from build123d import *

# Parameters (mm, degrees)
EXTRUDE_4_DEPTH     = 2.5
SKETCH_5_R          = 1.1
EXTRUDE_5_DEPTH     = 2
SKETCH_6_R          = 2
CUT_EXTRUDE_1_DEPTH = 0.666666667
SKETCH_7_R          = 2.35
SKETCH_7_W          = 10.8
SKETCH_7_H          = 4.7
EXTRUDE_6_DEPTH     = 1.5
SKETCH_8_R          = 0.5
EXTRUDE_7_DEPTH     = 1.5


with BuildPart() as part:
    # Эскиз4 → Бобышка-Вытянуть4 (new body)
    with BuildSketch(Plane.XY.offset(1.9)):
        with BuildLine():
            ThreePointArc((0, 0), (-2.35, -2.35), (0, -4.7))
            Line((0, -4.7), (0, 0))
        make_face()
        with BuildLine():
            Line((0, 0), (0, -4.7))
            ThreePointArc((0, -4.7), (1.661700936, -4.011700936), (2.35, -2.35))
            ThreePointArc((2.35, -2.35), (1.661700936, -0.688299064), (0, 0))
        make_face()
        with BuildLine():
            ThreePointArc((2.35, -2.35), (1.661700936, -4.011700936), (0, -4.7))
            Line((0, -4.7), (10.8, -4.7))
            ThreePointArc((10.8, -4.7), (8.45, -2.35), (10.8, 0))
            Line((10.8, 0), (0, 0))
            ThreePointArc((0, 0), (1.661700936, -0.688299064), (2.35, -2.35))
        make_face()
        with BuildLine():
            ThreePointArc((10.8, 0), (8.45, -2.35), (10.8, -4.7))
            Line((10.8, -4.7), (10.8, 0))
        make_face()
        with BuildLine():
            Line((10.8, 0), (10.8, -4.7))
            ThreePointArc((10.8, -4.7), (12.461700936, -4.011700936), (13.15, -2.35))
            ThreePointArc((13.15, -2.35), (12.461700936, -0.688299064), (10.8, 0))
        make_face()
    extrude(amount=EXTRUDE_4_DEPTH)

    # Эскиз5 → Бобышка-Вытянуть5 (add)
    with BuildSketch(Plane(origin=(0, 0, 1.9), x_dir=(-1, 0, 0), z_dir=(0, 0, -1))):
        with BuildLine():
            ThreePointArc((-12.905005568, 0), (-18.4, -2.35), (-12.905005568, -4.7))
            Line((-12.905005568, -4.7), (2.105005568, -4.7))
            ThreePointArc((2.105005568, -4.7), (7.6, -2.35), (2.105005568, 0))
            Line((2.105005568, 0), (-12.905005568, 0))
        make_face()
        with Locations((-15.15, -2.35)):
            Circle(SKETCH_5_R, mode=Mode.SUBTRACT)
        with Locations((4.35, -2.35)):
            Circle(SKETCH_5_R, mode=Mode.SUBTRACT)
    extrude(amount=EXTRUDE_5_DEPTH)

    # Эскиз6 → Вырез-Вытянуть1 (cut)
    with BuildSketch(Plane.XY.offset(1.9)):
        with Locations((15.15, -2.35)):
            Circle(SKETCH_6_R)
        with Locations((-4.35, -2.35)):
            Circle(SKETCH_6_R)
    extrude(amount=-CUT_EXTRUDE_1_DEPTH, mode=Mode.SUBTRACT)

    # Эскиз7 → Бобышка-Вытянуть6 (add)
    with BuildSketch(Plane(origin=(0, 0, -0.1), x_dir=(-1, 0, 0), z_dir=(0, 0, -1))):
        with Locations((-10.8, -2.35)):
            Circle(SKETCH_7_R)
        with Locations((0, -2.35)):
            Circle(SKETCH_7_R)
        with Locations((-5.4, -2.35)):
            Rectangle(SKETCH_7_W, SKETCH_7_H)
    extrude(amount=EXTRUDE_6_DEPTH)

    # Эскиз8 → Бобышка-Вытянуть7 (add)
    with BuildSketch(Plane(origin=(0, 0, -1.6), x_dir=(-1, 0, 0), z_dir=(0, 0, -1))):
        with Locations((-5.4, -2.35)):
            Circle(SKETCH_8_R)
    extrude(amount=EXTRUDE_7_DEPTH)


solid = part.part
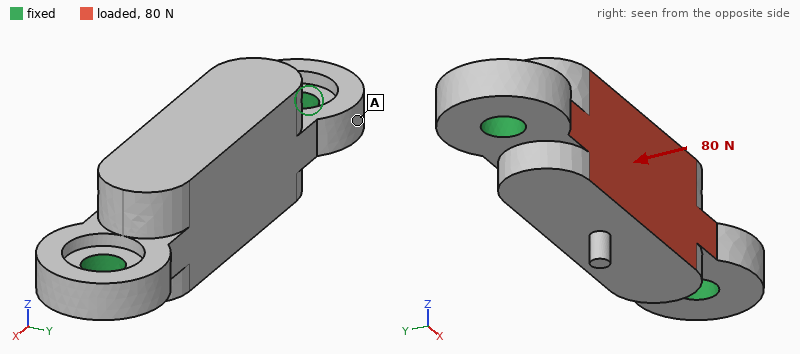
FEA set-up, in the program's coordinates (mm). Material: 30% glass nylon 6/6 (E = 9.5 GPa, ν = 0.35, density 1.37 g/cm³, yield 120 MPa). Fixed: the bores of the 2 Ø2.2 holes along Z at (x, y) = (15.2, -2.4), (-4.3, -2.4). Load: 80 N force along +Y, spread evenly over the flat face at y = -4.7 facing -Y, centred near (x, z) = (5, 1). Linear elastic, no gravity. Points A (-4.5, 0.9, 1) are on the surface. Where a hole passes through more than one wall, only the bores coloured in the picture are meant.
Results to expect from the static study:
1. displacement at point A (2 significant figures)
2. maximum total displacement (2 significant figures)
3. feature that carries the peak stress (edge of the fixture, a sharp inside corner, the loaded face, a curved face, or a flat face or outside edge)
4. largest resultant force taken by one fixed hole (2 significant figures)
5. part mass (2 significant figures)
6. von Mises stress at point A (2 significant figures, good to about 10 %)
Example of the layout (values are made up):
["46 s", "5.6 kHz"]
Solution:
["4.5 µm", "22 µm", "edge of the fixture", "40 N", "0.70 g", "3.9 MPa"]
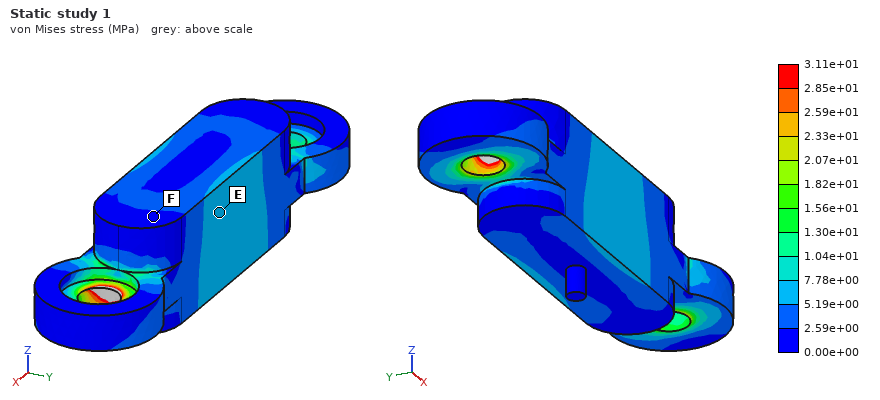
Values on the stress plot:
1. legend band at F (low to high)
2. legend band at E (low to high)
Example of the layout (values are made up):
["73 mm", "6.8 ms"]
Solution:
["0.00e+00 to 2.59e+00 MPa", "5.19e+00 to 7.78e+00 MPa"]
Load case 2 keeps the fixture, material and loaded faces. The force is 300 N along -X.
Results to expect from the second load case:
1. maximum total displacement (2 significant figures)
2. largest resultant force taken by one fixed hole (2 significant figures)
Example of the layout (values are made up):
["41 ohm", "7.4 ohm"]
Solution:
["12 µm", "160 N"]
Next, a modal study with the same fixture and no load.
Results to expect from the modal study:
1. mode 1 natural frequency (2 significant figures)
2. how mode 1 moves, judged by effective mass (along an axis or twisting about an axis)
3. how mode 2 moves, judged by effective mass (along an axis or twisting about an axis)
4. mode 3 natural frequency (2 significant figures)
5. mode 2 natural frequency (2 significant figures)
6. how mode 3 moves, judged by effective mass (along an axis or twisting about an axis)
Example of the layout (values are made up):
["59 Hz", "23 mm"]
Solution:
["14 kHz", "along Y", "along Z", "20 kHz", "18 kHz", "along Y"]
